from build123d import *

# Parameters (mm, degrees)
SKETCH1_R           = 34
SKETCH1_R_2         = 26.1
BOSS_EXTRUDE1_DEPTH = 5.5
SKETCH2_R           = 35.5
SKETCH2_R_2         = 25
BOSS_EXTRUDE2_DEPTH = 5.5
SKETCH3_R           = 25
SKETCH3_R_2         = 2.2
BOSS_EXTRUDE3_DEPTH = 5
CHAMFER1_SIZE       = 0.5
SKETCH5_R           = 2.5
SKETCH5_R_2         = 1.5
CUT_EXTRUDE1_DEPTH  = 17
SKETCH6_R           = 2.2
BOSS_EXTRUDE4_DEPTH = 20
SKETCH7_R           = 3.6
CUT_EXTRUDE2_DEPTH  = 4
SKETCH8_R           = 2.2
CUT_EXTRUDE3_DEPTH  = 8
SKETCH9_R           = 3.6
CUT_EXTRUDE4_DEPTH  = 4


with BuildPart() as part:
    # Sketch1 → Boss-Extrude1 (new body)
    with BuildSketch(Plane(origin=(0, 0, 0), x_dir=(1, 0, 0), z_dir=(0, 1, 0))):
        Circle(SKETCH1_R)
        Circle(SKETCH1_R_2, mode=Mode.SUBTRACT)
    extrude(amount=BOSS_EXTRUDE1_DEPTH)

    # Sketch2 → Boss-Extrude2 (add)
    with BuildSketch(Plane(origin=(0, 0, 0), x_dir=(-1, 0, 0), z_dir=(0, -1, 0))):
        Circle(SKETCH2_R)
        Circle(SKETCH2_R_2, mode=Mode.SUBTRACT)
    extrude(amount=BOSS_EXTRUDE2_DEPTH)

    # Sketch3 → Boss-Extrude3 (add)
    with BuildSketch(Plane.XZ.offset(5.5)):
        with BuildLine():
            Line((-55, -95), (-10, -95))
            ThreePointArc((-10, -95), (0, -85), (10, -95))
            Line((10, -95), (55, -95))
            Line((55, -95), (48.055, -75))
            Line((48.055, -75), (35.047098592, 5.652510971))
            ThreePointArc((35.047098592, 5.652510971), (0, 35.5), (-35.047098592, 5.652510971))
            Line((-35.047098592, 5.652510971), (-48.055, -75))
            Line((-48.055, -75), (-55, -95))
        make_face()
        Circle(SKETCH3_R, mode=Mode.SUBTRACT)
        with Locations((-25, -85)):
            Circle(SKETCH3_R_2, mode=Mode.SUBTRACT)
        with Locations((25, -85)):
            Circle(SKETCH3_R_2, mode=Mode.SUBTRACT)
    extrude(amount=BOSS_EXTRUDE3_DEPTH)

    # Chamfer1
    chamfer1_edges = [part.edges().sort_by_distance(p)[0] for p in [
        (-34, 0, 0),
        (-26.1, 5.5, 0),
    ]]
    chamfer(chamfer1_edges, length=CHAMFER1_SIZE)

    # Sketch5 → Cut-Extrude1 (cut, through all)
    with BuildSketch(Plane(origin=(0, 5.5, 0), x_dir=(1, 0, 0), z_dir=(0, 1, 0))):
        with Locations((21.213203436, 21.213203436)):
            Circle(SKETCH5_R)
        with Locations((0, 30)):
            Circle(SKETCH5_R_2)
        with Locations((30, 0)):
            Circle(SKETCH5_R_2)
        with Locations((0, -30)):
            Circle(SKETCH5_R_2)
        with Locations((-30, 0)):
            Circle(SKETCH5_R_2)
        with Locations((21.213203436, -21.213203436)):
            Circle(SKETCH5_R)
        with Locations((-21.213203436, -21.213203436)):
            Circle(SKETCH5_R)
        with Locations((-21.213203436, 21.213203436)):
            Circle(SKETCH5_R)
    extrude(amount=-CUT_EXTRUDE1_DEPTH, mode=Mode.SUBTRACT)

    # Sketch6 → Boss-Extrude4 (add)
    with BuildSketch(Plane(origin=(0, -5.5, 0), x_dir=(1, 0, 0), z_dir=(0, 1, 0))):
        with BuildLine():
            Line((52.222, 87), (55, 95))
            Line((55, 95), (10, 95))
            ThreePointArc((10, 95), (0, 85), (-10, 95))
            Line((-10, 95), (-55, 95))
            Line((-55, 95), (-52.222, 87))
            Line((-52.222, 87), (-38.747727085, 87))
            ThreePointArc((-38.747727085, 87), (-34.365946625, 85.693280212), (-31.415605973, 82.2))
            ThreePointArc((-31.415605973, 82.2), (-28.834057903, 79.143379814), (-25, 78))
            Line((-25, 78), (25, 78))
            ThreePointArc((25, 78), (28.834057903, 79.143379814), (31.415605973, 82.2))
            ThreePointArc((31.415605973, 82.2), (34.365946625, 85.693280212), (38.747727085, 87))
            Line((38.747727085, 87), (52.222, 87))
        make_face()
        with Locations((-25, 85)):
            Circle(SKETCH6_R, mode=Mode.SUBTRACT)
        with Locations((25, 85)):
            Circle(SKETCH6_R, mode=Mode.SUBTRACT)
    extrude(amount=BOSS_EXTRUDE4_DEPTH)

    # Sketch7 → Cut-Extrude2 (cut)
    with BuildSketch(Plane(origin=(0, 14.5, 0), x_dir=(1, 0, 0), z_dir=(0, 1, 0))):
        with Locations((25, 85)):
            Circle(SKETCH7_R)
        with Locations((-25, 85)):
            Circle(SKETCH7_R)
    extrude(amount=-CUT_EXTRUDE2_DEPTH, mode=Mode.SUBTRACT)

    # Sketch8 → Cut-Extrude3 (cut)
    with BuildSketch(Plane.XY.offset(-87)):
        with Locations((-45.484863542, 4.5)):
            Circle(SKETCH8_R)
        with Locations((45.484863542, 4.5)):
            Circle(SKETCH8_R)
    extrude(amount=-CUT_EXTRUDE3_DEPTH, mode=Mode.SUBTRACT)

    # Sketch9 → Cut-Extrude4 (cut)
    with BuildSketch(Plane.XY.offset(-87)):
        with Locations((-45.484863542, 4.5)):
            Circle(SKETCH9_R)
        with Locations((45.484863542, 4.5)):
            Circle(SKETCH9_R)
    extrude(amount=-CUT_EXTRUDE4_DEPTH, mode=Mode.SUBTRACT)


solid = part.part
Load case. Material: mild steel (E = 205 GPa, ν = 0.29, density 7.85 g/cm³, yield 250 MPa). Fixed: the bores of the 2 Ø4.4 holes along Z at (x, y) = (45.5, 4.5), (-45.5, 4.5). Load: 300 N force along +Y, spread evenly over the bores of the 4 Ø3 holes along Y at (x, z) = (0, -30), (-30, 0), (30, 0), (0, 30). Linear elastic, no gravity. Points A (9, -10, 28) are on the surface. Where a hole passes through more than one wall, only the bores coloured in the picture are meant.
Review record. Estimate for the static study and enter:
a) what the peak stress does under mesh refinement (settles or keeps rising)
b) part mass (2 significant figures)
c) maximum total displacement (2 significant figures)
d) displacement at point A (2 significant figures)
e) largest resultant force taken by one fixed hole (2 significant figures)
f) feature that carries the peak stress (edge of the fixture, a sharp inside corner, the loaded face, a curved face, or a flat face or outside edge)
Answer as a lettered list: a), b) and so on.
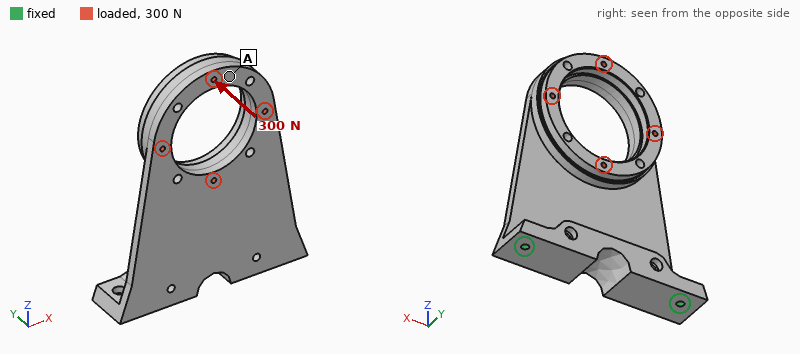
a) keeps rising
b) 650 g
c) 0.60 mm
d) 0.55 mm
e) 510 N
f) edge of the fixture
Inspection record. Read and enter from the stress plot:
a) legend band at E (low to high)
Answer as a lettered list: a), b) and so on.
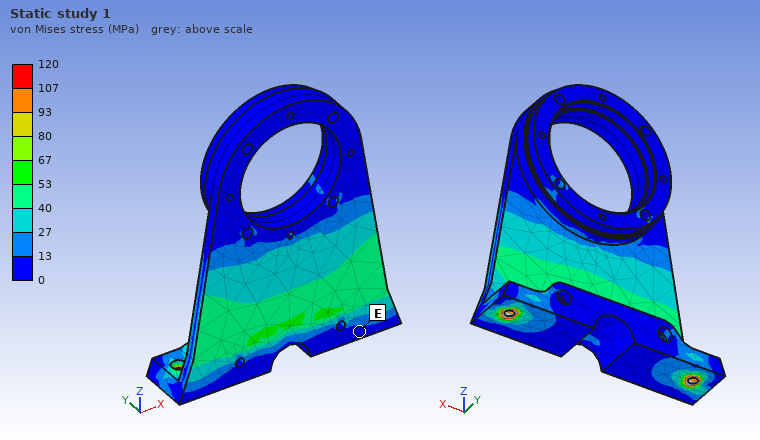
a) 0 to 13 MPa
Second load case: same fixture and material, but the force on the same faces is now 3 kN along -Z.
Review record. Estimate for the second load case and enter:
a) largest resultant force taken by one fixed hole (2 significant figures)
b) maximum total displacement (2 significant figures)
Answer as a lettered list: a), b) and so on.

a) 1.8 kN
b) 0.31 mm
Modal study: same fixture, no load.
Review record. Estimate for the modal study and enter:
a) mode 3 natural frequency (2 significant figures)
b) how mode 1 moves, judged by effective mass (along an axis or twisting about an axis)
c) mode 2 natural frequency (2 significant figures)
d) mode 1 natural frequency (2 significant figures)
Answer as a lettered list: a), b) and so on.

a) 1500 Hz
b) along Y
c) 1200 Hz
d) 270 Hz
